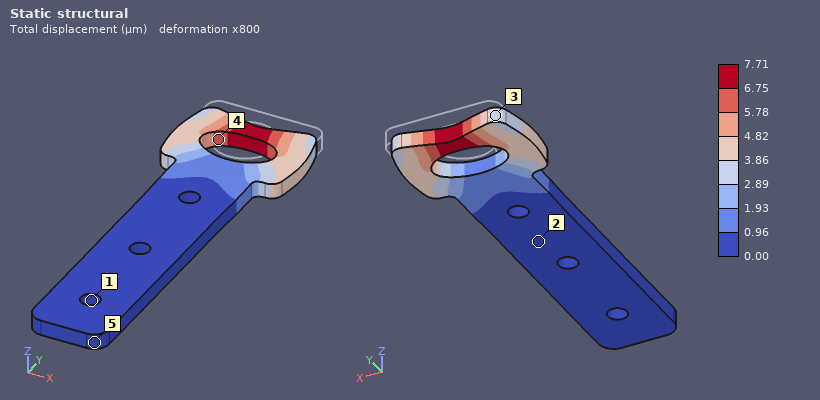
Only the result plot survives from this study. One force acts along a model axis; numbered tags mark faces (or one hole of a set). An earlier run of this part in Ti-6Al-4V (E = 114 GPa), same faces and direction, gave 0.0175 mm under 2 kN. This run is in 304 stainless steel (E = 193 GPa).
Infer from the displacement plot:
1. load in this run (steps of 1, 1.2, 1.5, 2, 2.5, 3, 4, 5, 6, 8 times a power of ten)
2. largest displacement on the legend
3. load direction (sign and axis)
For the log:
1.5 kN
7.71 µm
-Y
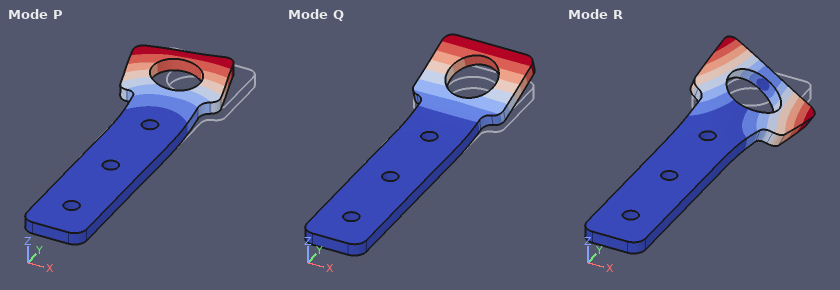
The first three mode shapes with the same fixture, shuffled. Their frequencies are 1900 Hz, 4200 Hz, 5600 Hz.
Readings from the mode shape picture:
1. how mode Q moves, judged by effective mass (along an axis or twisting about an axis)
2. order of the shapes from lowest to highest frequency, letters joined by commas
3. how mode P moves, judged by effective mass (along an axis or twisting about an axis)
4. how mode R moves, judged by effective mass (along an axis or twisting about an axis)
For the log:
along Z
Q, R, P
along X
twisting about Y
